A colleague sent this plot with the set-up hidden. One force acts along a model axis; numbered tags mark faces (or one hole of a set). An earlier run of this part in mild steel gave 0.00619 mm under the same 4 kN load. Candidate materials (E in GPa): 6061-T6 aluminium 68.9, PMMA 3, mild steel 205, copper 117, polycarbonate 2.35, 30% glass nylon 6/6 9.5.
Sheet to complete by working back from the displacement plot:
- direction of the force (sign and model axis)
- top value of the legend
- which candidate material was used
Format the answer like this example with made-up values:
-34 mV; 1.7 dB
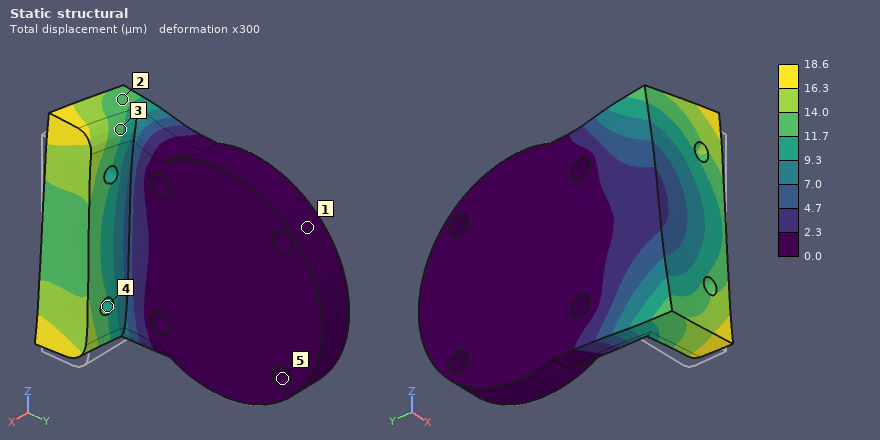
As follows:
+Z; 18.6 µm; 6061-T6 aluminium
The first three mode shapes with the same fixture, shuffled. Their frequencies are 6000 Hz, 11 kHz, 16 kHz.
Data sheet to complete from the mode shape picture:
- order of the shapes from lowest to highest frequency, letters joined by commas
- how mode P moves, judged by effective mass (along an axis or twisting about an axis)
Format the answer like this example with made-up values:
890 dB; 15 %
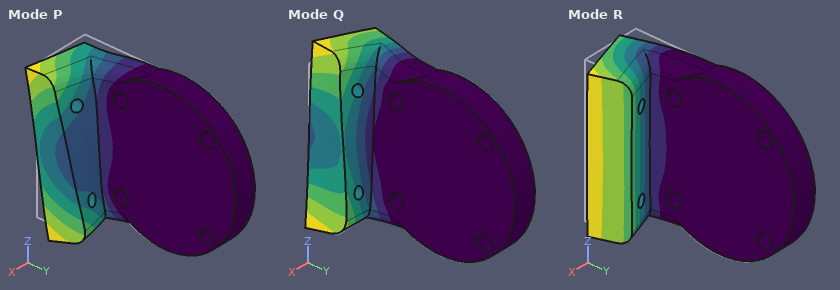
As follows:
R, Q, P; along Z
